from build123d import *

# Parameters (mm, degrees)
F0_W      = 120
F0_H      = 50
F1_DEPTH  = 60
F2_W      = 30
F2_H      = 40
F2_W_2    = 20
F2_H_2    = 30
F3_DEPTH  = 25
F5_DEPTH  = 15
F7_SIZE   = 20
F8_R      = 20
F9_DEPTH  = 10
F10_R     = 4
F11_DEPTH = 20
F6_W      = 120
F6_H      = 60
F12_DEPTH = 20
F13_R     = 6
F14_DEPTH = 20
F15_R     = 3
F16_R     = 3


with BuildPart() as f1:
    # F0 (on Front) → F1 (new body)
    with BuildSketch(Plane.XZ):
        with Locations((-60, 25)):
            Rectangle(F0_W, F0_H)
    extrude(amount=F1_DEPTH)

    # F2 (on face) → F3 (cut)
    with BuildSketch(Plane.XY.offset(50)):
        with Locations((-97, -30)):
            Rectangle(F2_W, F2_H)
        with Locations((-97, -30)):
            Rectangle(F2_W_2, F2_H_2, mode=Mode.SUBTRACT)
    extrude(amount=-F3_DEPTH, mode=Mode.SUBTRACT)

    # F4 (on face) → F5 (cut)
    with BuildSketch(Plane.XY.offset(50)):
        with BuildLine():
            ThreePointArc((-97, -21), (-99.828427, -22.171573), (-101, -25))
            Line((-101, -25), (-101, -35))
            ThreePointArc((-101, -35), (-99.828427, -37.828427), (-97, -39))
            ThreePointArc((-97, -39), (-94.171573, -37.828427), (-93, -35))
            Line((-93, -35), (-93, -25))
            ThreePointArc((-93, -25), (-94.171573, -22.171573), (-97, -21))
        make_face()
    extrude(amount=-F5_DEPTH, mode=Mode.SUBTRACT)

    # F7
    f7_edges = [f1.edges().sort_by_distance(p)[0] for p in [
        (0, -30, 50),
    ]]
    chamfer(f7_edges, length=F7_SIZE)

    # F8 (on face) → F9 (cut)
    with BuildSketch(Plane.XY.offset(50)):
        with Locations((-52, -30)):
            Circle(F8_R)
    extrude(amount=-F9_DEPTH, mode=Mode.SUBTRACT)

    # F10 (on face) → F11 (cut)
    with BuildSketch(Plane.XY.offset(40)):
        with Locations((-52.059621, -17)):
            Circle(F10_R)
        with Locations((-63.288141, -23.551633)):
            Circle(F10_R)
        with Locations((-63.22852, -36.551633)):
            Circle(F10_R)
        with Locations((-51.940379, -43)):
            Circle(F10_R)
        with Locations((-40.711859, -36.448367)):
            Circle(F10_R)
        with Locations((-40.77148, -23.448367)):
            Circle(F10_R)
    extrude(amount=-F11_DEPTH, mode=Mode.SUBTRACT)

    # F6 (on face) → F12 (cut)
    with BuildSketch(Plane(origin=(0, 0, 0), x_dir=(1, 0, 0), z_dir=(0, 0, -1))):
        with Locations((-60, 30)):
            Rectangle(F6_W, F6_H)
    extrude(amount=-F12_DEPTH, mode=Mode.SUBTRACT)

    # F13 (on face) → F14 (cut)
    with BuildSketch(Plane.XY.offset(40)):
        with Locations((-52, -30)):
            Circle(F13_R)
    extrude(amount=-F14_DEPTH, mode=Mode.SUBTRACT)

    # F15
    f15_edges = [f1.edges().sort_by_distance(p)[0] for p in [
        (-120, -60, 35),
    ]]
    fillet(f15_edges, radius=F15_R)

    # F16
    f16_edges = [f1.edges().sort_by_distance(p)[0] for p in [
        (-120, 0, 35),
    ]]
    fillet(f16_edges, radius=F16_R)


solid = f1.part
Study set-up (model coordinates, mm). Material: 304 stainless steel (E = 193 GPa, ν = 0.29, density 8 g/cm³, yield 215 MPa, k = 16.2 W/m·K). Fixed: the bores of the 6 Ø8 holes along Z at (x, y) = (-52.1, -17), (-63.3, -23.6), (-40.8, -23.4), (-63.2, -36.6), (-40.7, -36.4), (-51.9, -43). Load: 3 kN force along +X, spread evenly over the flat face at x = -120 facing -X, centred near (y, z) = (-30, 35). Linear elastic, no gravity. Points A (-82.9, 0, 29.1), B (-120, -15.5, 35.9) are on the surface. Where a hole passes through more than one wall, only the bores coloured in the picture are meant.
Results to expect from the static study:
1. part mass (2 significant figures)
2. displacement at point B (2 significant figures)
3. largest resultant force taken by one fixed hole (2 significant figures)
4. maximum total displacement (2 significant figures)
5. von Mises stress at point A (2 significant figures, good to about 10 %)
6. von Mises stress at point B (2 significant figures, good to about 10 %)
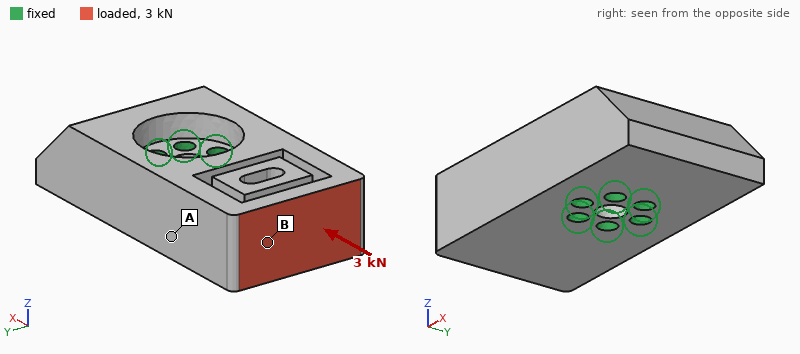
1.3 kg
3.8 µm
730 N
7.6 µm
2.9 MPa
9.2 MPa
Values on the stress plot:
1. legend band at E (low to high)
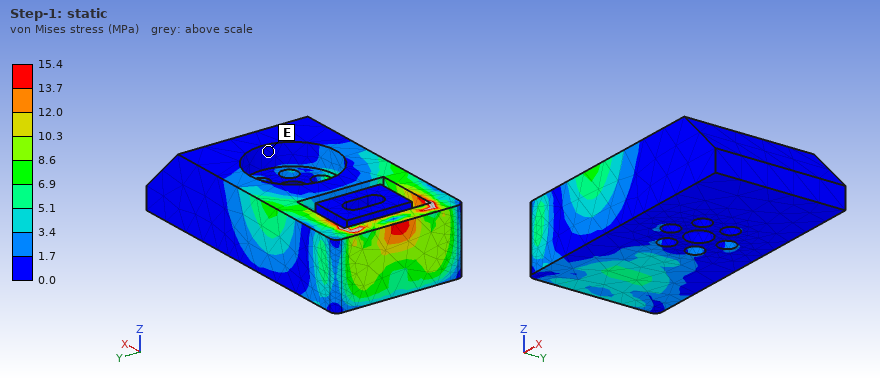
0.0 to 1.7 MPa
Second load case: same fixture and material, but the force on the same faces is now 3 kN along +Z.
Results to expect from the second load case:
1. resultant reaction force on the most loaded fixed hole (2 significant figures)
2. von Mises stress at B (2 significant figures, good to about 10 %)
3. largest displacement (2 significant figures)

2.5 kN
10 MPa
26 µm
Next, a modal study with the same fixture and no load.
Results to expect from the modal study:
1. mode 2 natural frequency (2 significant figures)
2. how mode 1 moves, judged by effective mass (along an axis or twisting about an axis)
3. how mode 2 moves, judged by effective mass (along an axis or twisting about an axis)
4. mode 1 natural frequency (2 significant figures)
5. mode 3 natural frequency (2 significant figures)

4800 Hz
along Z
along Y
4000 Hz
7600 Hz
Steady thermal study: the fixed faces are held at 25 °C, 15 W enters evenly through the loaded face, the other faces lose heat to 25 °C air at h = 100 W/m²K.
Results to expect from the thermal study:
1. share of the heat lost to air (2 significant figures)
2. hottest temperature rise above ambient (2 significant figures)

84 %
28 K
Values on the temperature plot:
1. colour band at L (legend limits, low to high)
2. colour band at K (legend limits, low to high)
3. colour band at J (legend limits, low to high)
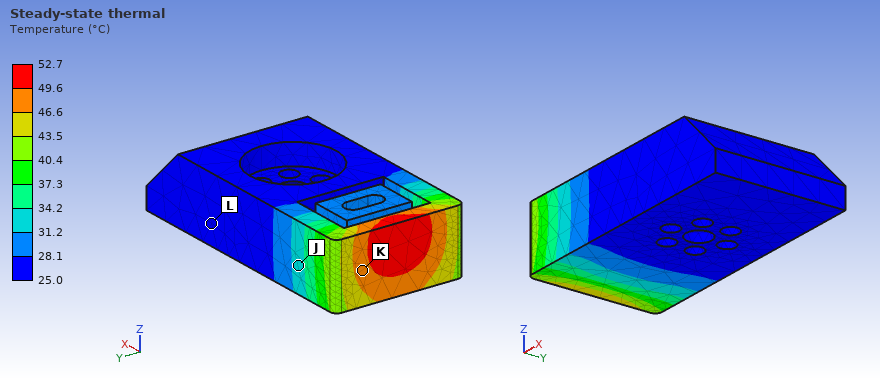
25.0 to 28.1 °C
46.6 to 49.6 °C
31.2 to 34.2 °C
